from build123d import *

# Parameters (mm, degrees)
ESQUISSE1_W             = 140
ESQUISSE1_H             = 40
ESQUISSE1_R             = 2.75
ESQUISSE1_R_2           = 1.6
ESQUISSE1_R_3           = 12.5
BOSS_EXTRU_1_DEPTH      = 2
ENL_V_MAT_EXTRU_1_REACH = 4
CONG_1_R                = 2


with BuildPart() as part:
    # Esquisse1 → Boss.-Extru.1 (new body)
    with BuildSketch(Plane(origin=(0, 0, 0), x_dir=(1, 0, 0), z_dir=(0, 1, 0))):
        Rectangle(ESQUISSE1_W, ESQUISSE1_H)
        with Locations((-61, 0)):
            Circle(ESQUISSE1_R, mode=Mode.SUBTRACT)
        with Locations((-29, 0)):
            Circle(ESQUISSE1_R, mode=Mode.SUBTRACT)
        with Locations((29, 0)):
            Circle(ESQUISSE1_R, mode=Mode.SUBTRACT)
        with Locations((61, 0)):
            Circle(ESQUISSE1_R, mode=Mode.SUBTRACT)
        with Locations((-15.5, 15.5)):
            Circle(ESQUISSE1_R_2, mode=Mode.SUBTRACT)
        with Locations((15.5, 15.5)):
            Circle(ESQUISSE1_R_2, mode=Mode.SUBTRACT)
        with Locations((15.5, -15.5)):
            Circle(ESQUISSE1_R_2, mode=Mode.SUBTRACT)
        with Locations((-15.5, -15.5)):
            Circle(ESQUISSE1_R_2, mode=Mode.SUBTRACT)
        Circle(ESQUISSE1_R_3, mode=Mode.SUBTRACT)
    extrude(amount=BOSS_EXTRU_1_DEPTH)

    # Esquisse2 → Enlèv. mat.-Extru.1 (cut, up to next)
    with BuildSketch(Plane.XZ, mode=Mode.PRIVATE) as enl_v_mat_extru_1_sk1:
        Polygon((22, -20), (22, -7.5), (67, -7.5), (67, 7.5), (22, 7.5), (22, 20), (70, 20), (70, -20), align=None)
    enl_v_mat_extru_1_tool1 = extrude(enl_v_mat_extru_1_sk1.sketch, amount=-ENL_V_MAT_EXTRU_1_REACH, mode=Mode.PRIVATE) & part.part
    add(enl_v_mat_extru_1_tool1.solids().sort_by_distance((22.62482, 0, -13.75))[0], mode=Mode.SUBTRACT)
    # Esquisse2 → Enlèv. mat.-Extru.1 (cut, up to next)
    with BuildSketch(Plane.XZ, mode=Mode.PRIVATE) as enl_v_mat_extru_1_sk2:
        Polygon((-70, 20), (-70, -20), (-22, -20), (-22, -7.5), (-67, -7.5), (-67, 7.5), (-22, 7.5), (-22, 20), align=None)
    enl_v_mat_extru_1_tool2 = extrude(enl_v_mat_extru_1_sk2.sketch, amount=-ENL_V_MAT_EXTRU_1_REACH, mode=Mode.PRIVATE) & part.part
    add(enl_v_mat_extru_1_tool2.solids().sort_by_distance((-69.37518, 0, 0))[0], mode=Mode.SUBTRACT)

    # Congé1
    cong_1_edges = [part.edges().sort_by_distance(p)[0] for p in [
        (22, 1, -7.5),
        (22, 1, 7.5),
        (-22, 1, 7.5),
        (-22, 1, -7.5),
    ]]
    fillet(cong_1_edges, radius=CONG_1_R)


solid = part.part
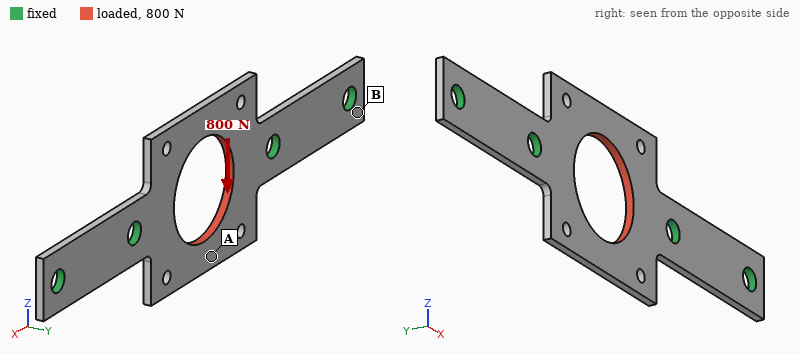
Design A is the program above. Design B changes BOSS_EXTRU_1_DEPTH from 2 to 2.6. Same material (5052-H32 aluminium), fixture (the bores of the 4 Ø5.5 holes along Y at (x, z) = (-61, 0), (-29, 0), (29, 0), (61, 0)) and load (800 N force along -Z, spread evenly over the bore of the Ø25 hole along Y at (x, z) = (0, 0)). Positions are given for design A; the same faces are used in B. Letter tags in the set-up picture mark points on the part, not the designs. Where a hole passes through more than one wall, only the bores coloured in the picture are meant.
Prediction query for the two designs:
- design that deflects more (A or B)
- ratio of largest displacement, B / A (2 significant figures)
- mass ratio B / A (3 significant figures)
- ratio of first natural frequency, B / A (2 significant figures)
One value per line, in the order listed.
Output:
A
0.77
1.30
1.3
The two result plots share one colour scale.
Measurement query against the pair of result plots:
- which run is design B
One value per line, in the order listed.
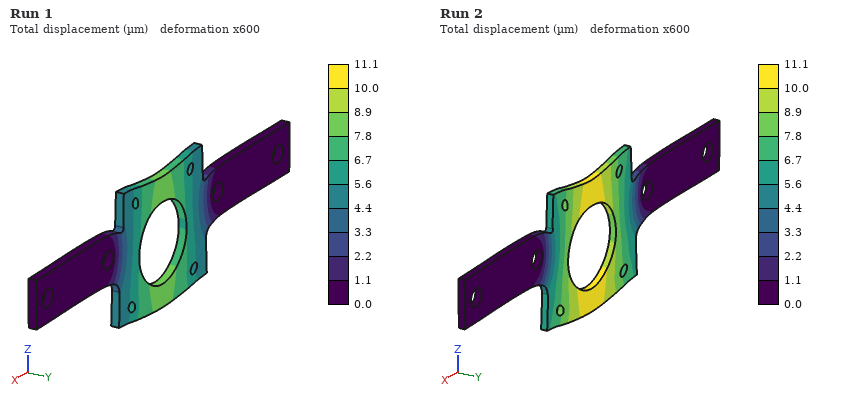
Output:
Run 1
